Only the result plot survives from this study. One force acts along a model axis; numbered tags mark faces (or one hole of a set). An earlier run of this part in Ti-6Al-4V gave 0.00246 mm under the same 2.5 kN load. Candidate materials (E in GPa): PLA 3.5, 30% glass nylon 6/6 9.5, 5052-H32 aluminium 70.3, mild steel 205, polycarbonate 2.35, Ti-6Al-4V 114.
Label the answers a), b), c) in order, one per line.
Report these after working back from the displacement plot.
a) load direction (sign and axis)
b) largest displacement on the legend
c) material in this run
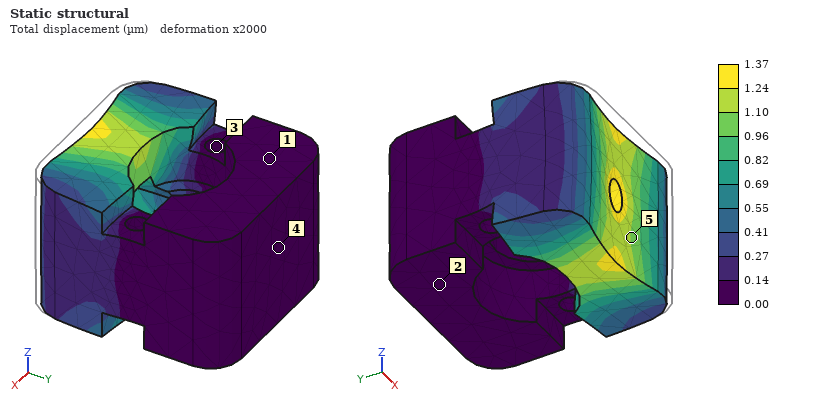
a) +Y
b) 1.37 µm
c) mild steel
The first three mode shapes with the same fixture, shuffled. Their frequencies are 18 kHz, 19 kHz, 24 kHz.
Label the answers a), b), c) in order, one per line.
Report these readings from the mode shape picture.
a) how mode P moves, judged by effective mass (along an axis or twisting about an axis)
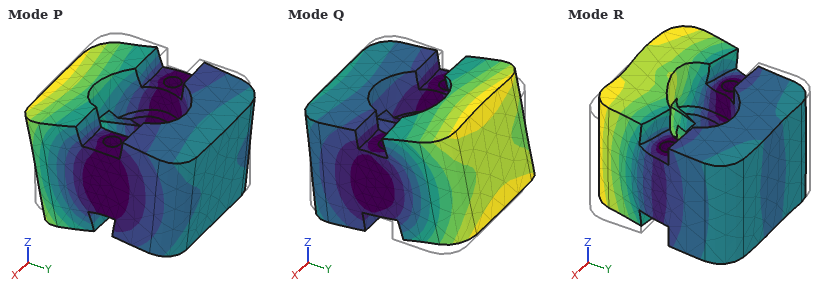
a) along Z
